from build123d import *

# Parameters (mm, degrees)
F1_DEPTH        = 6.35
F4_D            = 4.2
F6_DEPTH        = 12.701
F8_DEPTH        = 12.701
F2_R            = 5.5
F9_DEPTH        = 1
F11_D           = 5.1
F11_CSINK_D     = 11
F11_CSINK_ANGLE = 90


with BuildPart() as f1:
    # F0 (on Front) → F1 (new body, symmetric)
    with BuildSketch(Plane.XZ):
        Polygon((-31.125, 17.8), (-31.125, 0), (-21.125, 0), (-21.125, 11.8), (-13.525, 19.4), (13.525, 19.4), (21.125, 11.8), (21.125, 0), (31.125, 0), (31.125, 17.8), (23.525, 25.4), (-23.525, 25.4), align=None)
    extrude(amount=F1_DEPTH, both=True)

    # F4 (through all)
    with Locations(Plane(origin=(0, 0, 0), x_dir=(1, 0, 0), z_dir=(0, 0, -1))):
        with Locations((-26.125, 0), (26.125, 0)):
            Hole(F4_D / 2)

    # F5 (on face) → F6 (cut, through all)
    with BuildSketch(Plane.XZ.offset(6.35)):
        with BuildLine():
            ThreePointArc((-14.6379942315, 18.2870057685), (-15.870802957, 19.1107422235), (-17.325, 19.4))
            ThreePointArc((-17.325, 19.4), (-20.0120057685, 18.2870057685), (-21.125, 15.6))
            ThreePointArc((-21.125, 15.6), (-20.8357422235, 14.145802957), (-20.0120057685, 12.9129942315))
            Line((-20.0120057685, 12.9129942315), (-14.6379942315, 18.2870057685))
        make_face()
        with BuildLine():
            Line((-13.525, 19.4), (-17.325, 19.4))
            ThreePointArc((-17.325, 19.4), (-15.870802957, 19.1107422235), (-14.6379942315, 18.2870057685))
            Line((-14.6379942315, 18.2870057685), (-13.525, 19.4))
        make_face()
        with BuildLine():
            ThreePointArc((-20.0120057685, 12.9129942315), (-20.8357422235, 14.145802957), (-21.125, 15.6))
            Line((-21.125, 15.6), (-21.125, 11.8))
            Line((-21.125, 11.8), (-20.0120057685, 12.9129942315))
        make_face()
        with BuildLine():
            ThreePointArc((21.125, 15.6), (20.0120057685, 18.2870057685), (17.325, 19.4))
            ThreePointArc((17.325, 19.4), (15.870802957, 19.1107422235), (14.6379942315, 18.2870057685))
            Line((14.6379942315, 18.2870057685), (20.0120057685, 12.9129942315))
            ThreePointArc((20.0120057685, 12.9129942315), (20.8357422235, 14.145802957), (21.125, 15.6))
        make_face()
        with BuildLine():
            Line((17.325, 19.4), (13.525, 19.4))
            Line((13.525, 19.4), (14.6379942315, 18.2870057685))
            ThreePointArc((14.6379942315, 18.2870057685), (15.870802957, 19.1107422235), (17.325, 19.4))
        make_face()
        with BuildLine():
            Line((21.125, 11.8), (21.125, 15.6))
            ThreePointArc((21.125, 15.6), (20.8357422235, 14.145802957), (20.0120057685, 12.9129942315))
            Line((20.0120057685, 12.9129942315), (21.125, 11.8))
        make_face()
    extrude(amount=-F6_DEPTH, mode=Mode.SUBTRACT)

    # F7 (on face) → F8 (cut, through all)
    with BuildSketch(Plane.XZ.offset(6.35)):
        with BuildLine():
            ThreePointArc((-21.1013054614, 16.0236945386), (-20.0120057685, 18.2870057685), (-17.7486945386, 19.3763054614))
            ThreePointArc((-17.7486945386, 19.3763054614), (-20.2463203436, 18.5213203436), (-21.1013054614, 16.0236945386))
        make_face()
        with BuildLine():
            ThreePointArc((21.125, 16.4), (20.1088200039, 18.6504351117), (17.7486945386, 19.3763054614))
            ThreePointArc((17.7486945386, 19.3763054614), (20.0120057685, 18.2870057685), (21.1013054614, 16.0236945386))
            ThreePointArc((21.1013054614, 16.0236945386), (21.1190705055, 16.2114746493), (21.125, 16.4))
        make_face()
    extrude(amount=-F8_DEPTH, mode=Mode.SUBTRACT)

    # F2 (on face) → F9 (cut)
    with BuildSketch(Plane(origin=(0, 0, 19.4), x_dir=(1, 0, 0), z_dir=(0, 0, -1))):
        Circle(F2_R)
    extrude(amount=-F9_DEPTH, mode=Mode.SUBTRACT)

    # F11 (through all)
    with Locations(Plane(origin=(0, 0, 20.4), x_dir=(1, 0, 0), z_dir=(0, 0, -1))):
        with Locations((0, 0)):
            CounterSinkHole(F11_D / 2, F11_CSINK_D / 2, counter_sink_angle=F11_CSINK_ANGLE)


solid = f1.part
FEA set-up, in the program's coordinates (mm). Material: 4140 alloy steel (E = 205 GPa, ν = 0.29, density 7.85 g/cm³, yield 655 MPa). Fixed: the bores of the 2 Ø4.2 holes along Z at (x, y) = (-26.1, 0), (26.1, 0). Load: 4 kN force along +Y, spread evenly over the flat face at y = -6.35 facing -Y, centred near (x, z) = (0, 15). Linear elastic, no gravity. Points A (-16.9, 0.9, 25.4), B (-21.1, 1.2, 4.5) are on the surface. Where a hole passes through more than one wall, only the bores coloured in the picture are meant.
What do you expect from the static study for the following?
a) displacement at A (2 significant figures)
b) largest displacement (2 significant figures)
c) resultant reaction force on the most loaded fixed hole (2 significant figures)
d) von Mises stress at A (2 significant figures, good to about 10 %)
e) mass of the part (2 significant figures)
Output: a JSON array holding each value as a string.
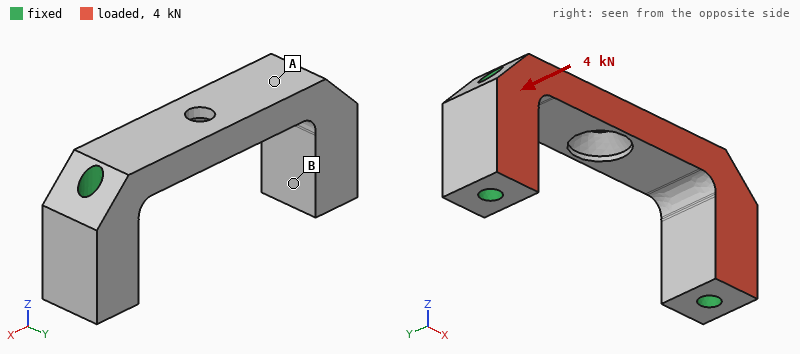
["2.7 µm", "7.2 µm", "2.0 kN", "17 MPa", "63 g"]
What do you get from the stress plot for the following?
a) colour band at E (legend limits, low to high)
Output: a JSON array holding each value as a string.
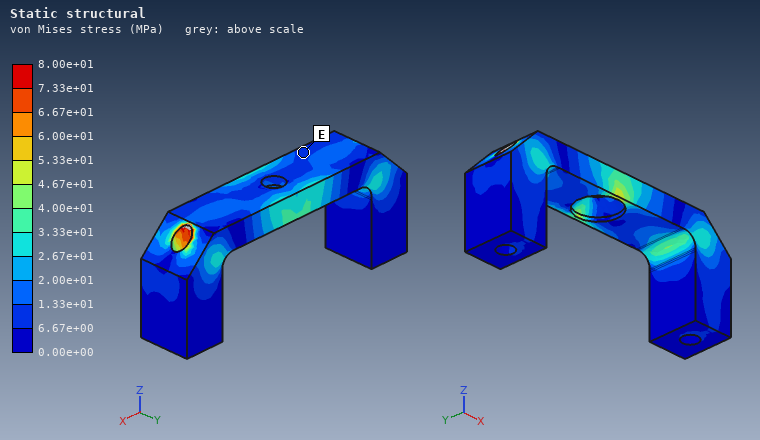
["6.67e+00 to 1.33e+01 MPa"]
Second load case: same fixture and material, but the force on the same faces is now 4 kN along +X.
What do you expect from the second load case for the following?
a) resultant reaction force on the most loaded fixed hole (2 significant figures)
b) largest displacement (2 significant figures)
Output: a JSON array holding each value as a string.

["2.0 kN", "1.7 µm"]
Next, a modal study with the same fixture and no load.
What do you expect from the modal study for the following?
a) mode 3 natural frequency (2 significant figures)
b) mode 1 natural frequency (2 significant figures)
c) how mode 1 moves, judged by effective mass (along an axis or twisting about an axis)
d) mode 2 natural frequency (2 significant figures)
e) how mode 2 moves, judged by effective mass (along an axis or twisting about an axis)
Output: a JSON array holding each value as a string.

["28 kHz", "14 kHz", "along Z", "18 kHz", "along Y"]
